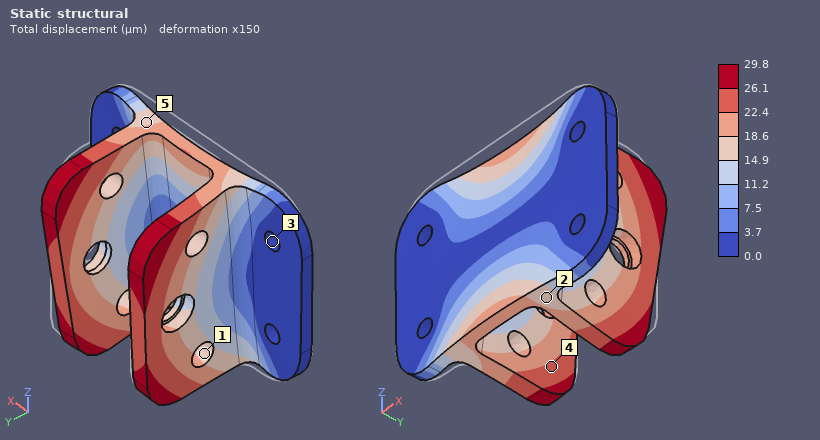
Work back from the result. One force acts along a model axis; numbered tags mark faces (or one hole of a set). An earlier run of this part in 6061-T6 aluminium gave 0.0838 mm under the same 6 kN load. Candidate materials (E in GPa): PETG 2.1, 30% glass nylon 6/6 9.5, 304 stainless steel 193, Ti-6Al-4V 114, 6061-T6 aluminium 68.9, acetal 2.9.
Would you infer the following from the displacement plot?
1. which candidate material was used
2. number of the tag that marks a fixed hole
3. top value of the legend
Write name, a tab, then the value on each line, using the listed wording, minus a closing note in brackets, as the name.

which candidate material was used	304 stainless steel
number of the tag that marks a fixed hole	3
top value of the legend	29.8 µm
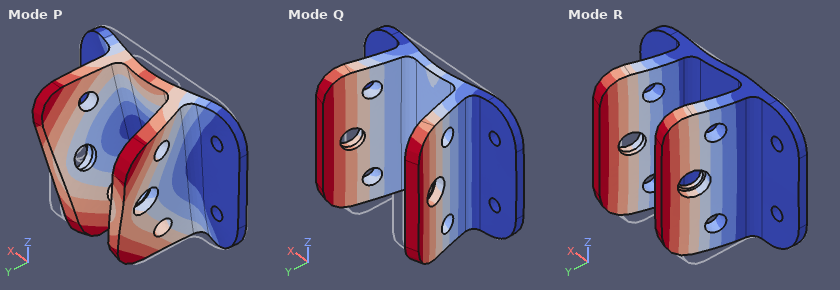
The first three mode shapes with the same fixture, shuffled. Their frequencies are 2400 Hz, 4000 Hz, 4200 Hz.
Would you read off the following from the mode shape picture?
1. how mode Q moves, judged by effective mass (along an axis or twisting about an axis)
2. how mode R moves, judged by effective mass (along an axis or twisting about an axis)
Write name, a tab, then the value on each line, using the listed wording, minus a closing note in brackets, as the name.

how mode Q moves, judged by effective mass	along Y
how mode R moves, judged by effective mass	along X
